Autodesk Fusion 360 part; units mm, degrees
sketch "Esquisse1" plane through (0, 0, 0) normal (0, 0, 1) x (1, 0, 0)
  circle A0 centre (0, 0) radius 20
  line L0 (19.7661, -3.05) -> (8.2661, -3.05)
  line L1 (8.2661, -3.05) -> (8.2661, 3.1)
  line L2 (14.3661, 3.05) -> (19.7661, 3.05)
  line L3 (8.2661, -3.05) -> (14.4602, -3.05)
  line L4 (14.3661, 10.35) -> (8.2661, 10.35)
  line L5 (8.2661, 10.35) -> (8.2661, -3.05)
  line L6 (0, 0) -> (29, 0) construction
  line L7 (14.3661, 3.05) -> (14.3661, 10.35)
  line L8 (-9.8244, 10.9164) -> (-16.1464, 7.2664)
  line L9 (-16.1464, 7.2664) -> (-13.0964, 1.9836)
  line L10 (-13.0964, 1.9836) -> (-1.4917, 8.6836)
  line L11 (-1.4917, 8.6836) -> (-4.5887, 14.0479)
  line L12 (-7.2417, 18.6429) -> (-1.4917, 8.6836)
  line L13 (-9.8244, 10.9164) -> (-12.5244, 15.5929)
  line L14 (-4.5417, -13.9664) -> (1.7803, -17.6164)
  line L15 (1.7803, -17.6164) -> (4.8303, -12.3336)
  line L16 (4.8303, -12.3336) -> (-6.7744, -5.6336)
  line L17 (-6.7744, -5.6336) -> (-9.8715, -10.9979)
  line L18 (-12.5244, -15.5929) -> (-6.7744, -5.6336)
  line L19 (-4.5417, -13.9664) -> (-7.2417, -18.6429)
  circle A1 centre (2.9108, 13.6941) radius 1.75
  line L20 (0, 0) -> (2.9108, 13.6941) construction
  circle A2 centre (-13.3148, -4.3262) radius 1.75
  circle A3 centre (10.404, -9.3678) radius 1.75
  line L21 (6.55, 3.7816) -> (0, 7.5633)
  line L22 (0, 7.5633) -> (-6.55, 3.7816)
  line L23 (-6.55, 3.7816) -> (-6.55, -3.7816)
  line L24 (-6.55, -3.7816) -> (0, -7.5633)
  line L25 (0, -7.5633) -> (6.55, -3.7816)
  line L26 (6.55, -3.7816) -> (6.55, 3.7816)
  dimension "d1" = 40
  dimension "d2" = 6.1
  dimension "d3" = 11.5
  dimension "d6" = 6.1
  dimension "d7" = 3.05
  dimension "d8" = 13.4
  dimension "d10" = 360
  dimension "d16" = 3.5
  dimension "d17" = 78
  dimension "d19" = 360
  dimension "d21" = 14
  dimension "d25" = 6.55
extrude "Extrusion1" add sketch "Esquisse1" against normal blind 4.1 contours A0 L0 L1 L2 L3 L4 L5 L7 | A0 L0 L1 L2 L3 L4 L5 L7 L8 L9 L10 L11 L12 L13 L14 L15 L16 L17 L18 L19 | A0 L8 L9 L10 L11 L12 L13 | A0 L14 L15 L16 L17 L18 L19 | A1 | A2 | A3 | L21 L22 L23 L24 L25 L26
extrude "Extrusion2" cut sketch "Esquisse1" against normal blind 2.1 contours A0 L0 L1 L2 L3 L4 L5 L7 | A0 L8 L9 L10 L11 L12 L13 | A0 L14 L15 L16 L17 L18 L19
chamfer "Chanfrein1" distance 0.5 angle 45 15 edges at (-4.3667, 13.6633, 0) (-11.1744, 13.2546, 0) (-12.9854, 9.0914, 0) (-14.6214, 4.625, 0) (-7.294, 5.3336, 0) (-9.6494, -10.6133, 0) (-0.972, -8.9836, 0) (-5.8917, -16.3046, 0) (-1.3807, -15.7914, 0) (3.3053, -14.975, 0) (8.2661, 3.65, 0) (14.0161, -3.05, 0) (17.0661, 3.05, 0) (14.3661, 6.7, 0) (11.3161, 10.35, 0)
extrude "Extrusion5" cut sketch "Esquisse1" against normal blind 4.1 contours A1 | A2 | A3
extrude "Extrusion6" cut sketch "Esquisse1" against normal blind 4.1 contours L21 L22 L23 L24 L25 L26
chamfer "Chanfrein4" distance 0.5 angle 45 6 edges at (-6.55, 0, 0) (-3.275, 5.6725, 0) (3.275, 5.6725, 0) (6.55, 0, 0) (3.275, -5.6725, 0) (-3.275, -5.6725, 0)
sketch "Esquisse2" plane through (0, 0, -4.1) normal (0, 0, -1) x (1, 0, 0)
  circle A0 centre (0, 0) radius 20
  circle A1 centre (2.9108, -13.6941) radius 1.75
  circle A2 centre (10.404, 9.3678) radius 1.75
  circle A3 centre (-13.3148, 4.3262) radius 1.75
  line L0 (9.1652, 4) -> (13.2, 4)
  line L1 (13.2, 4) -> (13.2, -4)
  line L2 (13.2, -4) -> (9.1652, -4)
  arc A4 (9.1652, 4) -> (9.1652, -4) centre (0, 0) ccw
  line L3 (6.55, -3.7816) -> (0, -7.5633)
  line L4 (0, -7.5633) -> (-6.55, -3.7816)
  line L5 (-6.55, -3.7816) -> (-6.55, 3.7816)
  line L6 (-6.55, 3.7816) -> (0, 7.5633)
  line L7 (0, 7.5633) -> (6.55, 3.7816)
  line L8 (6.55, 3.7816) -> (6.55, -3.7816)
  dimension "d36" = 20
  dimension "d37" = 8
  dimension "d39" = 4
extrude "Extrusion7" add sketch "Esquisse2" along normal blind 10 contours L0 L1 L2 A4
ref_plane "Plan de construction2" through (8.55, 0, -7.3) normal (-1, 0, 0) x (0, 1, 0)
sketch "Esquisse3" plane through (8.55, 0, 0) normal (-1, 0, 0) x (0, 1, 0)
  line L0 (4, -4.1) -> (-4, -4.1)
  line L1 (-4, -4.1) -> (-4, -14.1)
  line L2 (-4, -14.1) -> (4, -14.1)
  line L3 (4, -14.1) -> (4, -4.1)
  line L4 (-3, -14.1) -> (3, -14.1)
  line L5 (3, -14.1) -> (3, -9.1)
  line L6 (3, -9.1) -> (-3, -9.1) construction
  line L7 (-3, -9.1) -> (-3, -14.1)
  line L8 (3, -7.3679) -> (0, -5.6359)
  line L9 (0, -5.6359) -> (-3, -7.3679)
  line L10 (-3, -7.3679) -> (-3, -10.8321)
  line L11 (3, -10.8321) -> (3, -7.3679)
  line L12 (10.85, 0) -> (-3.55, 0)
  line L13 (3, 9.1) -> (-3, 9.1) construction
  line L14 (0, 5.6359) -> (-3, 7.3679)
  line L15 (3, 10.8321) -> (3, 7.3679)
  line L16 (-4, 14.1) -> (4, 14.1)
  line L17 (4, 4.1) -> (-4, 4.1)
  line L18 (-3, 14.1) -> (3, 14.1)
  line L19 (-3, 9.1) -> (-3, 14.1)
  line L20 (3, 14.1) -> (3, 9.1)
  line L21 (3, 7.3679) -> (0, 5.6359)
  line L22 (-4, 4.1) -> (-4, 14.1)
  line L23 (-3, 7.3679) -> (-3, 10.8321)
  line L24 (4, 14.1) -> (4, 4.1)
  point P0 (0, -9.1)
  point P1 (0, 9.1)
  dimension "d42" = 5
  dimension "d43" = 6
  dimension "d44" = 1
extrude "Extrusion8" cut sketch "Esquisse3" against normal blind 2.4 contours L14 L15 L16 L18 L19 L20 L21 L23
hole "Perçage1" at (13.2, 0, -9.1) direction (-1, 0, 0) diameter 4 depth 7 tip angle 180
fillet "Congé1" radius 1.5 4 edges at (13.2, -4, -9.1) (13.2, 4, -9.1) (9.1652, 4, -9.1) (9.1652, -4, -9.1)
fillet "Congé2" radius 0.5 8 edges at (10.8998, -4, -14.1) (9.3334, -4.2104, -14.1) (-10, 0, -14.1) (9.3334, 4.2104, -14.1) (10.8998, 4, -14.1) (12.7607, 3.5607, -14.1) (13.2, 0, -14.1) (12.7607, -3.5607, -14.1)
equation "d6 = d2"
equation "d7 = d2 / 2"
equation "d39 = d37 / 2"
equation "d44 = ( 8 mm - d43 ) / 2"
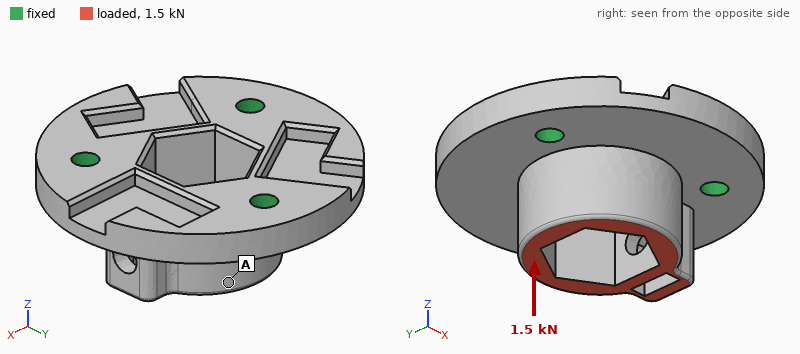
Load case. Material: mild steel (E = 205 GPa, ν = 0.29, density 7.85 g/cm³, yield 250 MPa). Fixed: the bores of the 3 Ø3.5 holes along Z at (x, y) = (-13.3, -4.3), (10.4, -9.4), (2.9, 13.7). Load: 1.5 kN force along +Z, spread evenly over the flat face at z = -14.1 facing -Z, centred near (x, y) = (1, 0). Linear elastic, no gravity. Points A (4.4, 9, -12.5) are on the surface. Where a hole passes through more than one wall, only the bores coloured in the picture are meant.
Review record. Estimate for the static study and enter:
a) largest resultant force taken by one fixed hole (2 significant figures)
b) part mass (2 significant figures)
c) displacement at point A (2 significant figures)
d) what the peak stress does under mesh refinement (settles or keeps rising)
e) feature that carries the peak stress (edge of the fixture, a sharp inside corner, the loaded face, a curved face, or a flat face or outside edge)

590 N
43 g
1.9 µm
keeps rising
edge of the fixture
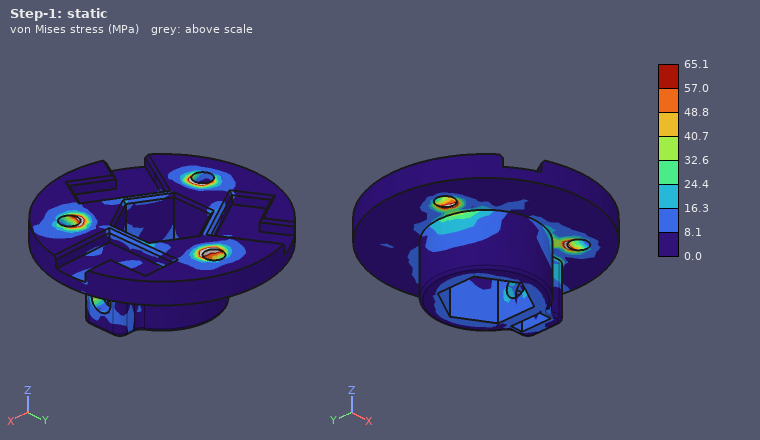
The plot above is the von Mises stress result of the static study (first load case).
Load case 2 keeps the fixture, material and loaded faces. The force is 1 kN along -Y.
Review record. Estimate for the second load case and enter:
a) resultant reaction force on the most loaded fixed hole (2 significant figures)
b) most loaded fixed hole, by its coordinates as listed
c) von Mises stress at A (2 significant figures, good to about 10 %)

710 N
(2.9, 13.7)
18 MPa
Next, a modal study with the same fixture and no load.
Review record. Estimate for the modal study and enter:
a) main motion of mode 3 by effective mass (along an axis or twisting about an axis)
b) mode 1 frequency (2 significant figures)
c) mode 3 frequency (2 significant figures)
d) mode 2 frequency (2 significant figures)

along Z
18 kHz
21 kHz
19 kHz
